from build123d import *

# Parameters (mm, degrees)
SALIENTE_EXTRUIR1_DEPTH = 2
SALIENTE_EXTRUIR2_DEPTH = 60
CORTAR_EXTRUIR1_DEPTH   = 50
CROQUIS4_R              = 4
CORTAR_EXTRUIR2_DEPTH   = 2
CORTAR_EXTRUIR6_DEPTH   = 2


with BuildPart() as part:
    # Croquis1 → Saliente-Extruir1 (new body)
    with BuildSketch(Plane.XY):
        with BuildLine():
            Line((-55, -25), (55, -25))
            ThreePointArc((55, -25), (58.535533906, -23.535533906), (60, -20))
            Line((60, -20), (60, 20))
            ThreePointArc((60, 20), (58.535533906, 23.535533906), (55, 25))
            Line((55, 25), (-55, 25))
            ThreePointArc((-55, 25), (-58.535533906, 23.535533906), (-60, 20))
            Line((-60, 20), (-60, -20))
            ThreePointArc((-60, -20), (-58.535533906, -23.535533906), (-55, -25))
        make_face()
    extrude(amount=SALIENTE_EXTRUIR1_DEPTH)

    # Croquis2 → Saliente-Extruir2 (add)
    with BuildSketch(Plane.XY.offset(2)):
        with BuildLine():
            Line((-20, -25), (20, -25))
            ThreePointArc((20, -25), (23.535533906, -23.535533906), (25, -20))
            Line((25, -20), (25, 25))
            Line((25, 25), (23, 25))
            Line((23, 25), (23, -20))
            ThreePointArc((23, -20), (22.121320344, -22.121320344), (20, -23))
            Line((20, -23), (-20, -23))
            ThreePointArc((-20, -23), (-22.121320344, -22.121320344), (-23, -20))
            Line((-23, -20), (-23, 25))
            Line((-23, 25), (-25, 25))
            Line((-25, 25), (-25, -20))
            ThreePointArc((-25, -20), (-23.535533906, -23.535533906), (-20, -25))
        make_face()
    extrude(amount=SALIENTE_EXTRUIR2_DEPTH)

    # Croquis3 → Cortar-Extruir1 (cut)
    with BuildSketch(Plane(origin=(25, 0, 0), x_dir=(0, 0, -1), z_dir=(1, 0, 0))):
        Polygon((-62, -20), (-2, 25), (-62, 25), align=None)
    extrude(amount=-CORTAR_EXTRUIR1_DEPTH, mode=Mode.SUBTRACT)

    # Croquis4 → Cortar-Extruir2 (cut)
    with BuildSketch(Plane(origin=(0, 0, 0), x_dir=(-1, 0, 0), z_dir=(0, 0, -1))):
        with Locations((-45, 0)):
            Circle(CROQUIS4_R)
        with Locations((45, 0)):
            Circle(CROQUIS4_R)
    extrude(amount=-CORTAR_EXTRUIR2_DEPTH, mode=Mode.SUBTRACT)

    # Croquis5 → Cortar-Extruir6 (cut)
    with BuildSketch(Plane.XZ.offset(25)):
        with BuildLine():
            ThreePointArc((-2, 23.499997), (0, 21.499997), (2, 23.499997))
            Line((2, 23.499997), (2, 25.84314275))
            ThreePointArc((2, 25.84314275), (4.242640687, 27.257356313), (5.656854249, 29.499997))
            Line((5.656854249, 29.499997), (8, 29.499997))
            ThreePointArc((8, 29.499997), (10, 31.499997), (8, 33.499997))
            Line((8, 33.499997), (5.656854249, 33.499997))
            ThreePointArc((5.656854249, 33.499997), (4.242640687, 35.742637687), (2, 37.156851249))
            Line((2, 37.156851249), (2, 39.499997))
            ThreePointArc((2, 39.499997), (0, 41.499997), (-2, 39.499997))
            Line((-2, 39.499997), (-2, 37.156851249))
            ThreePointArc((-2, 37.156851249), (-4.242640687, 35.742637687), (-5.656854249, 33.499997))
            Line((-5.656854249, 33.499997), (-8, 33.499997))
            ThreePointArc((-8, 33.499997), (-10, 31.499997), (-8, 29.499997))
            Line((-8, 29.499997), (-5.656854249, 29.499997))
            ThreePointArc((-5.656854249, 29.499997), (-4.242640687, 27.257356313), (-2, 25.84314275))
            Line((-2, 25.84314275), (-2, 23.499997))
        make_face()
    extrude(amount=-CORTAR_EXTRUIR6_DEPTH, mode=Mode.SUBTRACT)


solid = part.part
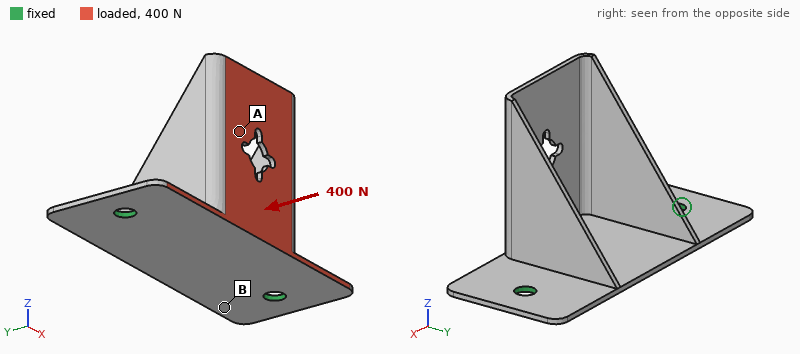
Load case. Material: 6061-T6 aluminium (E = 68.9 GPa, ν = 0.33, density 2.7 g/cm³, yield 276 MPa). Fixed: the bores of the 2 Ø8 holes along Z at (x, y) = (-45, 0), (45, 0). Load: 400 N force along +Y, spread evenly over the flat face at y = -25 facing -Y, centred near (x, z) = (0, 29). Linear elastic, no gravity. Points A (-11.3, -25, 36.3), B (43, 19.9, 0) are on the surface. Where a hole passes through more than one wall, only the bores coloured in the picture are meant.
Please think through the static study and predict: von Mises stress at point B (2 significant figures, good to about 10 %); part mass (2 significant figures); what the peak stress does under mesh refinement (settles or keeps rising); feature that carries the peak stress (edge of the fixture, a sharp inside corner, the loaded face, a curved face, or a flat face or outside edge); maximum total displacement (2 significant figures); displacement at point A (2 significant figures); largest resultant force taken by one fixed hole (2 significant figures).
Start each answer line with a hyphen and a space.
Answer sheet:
- 56 MPa
- 62 g
- keeps rising
- edge of the fixture
- 1.6 mm
- 0.98 mm
- 200 N
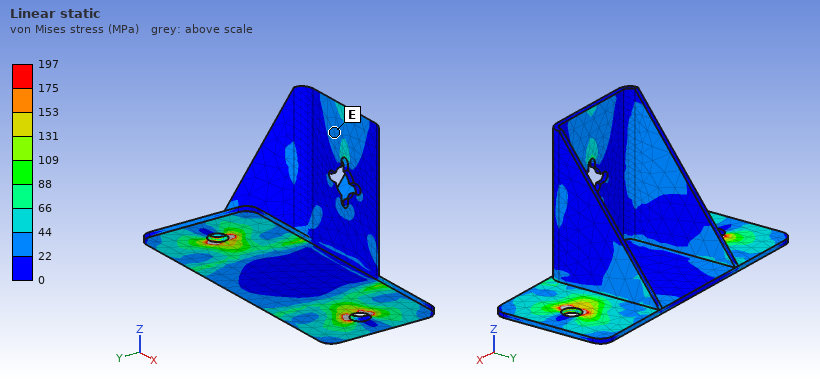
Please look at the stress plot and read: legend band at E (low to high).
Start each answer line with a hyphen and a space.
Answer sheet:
- 22 to 44 MPa
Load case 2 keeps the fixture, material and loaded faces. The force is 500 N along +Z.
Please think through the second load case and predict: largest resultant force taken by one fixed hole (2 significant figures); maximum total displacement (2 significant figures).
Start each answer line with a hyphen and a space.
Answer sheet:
- 270 N
- 1.5 mm
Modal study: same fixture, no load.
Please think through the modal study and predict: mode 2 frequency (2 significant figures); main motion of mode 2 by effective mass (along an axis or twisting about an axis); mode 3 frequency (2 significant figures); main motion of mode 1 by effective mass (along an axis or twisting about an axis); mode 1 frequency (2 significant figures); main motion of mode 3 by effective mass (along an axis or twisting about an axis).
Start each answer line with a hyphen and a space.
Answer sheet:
- 990 Hz
- along X
- 1300 Hz
- along Y
- 540 Hz
- along Z
